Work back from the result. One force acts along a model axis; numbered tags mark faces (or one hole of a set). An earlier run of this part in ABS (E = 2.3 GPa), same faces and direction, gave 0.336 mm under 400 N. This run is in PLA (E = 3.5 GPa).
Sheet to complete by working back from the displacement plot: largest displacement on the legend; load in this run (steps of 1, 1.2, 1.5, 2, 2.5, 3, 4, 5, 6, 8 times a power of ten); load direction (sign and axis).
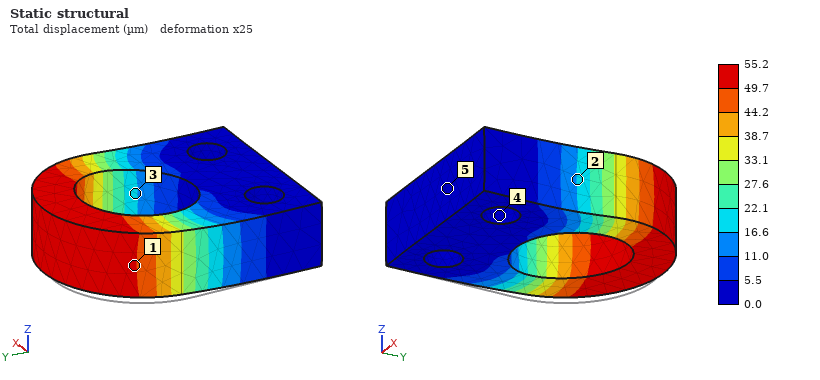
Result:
55.2 µm
100 N
+X
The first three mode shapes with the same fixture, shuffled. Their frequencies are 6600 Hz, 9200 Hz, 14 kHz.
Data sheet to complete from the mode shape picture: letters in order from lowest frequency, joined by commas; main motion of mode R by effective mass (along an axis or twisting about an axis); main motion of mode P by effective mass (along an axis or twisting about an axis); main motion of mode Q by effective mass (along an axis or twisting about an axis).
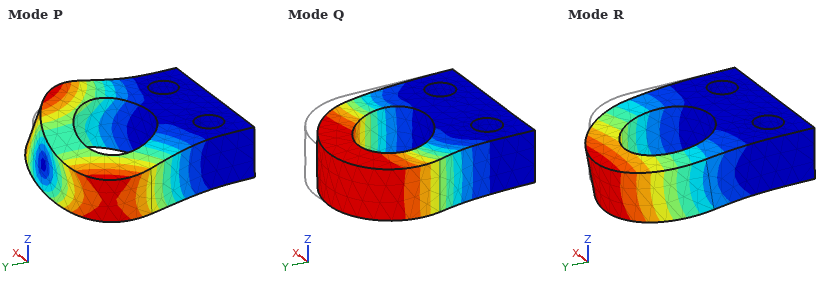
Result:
R, Q, P
along Z
twisting about Y
along X
